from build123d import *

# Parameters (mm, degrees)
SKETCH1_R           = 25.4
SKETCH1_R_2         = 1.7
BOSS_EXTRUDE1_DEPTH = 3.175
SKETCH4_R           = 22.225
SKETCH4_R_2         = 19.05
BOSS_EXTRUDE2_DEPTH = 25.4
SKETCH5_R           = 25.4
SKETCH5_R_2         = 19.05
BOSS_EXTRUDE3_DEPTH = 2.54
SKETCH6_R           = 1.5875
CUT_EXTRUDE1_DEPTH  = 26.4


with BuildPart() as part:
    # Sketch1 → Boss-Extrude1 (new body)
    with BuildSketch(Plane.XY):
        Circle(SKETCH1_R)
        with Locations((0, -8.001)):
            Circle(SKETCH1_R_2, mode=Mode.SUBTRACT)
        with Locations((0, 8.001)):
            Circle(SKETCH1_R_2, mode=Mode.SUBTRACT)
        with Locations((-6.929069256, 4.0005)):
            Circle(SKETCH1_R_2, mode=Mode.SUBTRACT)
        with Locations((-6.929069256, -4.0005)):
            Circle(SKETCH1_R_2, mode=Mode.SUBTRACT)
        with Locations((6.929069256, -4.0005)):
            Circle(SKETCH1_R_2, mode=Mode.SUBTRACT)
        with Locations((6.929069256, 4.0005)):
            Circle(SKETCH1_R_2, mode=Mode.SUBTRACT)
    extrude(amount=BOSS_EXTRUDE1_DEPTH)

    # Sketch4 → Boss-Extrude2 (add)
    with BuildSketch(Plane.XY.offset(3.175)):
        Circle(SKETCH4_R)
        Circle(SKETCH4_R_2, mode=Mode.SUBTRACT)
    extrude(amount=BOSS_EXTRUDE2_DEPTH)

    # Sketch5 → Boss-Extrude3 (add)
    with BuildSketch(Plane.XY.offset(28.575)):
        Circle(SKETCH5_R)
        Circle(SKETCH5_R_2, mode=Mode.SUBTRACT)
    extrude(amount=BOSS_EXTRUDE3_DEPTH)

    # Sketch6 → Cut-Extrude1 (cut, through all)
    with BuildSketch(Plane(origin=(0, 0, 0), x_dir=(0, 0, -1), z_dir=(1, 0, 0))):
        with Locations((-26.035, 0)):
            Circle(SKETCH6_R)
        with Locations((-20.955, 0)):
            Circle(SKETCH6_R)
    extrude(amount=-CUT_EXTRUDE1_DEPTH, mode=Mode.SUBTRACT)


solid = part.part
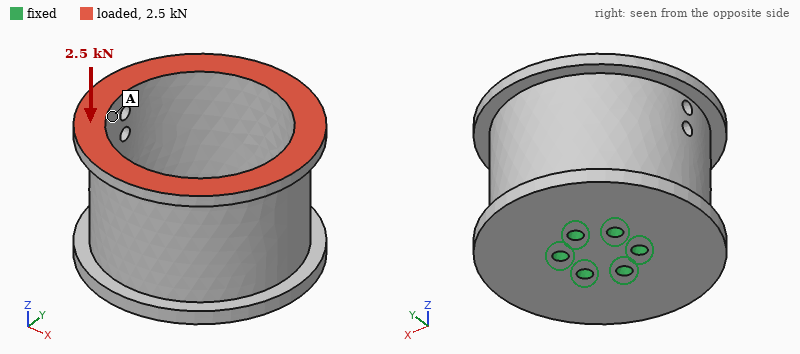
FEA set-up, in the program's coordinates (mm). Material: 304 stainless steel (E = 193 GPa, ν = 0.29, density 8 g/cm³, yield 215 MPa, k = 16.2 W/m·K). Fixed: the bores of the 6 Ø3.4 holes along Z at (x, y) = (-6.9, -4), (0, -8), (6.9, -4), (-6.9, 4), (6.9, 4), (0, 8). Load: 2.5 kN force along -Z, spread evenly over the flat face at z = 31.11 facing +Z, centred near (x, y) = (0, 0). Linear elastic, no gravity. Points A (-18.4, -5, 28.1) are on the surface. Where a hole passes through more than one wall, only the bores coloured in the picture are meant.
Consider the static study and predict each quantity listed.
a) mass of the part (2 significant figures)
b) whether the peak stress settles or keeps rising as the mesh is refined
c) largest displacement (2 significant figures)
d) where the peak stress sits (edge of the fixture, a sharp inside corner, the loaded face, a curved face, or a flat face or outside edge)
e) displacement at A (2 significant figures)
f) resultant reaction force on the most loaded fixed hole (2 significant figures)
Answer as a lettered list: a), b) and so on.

a) 150 g
b) keeps rising
c) 13 µm
d) edge of the fixture
e) 11 µm
f) 440 N
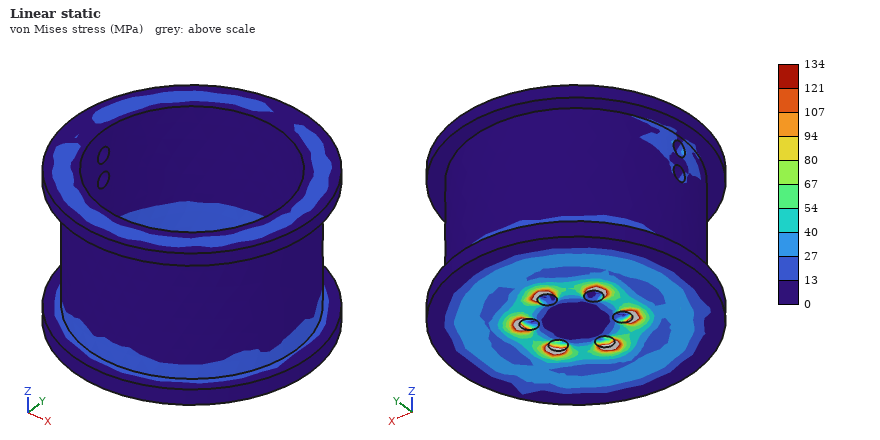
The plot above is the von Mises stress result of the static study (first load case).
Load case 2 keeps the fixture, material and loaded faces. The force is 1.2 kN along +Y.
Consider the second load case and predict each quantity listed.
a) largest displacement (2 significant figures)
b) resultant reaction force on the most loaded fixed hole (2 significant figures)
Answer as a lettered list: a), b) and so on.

a) 54 µm
b) 810 N
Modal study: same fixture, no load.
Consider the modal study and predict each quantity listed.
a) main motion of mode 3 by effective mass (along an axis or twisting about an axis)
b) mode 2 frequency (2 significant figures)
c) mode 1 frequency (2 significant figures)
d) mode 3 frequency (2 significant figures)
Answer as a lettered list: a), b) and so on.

a) along Z
b) 3200 Hz
c) 3200 Hz
d) 6600 Hz
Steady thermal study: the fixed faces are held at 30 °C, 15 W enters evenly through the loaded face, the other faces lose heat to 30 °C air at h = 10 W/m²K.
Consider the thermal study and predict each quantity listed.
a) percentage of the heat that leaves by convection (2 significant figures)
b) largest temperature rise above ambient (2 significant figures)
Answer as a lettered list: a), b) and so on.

a) 33 %
b) 81 K
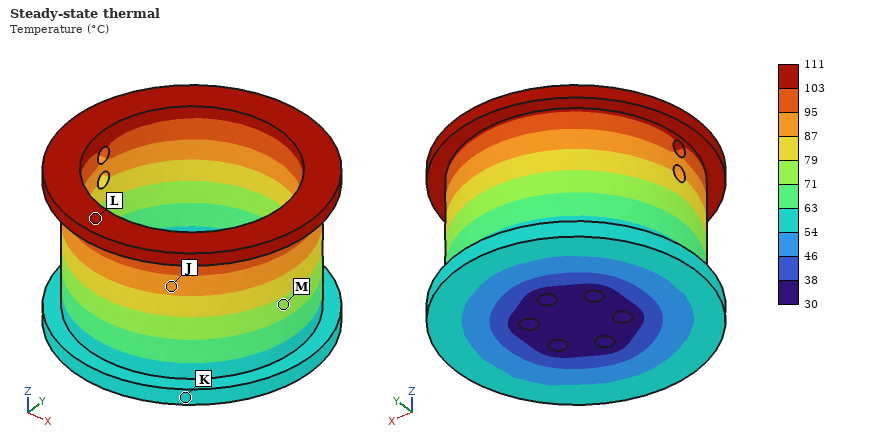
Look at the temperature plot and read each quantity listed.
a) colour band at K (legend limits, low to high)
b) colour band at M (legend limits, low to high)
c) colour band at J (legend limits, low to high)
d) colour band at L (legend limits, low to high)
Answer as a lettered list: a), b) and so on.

a) 54 to 63 °C
b) 71 to 79 °C
c) 87 to 95 °C
d) 103 to 111 °C
